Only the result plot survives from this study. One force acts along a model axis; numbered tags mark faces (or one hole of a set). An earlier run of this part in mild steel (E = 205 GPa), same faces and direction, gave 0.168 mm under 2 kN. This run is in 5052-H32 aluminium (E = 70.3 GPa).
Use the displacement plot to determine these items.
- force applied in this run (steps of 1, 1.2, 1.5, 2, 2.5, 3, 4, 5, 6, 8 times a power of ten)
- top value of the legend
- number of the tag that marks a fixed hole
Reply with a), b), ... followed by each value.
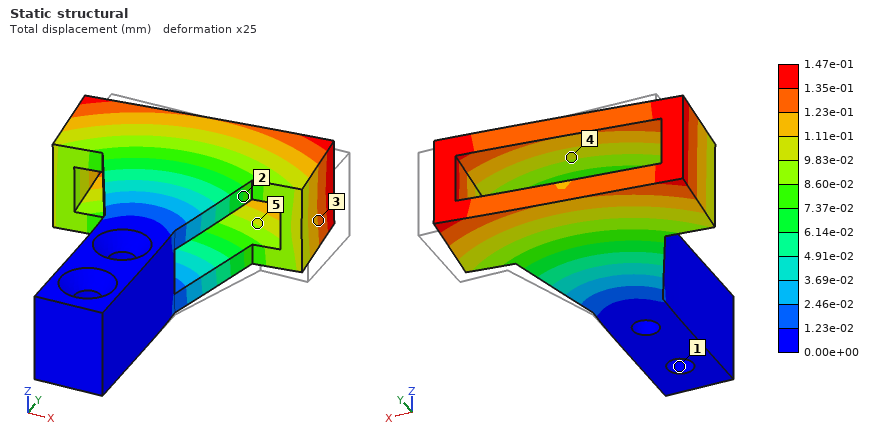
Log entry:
a) 600 N
b) 1.47e-01 mm
c) 1
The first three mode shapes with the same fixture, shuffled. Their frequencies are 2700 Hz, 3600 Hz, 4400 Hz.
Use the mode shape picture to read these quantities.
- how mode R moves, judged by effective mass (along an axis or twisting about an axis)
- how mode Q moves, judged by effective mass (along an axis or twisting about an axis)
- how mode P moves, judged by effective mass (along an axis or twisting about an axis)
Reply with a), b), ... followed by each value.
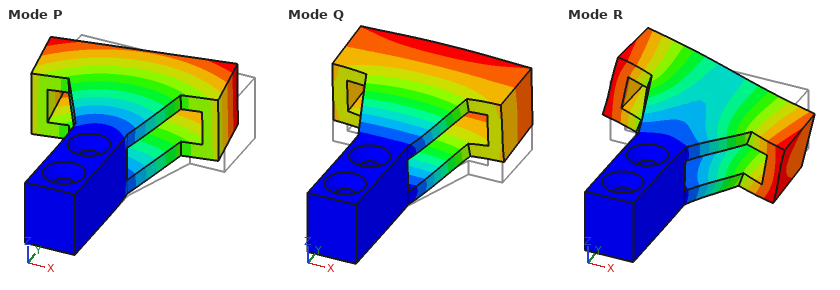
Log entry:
a) twisting about Y
b) along Z
c) along X
